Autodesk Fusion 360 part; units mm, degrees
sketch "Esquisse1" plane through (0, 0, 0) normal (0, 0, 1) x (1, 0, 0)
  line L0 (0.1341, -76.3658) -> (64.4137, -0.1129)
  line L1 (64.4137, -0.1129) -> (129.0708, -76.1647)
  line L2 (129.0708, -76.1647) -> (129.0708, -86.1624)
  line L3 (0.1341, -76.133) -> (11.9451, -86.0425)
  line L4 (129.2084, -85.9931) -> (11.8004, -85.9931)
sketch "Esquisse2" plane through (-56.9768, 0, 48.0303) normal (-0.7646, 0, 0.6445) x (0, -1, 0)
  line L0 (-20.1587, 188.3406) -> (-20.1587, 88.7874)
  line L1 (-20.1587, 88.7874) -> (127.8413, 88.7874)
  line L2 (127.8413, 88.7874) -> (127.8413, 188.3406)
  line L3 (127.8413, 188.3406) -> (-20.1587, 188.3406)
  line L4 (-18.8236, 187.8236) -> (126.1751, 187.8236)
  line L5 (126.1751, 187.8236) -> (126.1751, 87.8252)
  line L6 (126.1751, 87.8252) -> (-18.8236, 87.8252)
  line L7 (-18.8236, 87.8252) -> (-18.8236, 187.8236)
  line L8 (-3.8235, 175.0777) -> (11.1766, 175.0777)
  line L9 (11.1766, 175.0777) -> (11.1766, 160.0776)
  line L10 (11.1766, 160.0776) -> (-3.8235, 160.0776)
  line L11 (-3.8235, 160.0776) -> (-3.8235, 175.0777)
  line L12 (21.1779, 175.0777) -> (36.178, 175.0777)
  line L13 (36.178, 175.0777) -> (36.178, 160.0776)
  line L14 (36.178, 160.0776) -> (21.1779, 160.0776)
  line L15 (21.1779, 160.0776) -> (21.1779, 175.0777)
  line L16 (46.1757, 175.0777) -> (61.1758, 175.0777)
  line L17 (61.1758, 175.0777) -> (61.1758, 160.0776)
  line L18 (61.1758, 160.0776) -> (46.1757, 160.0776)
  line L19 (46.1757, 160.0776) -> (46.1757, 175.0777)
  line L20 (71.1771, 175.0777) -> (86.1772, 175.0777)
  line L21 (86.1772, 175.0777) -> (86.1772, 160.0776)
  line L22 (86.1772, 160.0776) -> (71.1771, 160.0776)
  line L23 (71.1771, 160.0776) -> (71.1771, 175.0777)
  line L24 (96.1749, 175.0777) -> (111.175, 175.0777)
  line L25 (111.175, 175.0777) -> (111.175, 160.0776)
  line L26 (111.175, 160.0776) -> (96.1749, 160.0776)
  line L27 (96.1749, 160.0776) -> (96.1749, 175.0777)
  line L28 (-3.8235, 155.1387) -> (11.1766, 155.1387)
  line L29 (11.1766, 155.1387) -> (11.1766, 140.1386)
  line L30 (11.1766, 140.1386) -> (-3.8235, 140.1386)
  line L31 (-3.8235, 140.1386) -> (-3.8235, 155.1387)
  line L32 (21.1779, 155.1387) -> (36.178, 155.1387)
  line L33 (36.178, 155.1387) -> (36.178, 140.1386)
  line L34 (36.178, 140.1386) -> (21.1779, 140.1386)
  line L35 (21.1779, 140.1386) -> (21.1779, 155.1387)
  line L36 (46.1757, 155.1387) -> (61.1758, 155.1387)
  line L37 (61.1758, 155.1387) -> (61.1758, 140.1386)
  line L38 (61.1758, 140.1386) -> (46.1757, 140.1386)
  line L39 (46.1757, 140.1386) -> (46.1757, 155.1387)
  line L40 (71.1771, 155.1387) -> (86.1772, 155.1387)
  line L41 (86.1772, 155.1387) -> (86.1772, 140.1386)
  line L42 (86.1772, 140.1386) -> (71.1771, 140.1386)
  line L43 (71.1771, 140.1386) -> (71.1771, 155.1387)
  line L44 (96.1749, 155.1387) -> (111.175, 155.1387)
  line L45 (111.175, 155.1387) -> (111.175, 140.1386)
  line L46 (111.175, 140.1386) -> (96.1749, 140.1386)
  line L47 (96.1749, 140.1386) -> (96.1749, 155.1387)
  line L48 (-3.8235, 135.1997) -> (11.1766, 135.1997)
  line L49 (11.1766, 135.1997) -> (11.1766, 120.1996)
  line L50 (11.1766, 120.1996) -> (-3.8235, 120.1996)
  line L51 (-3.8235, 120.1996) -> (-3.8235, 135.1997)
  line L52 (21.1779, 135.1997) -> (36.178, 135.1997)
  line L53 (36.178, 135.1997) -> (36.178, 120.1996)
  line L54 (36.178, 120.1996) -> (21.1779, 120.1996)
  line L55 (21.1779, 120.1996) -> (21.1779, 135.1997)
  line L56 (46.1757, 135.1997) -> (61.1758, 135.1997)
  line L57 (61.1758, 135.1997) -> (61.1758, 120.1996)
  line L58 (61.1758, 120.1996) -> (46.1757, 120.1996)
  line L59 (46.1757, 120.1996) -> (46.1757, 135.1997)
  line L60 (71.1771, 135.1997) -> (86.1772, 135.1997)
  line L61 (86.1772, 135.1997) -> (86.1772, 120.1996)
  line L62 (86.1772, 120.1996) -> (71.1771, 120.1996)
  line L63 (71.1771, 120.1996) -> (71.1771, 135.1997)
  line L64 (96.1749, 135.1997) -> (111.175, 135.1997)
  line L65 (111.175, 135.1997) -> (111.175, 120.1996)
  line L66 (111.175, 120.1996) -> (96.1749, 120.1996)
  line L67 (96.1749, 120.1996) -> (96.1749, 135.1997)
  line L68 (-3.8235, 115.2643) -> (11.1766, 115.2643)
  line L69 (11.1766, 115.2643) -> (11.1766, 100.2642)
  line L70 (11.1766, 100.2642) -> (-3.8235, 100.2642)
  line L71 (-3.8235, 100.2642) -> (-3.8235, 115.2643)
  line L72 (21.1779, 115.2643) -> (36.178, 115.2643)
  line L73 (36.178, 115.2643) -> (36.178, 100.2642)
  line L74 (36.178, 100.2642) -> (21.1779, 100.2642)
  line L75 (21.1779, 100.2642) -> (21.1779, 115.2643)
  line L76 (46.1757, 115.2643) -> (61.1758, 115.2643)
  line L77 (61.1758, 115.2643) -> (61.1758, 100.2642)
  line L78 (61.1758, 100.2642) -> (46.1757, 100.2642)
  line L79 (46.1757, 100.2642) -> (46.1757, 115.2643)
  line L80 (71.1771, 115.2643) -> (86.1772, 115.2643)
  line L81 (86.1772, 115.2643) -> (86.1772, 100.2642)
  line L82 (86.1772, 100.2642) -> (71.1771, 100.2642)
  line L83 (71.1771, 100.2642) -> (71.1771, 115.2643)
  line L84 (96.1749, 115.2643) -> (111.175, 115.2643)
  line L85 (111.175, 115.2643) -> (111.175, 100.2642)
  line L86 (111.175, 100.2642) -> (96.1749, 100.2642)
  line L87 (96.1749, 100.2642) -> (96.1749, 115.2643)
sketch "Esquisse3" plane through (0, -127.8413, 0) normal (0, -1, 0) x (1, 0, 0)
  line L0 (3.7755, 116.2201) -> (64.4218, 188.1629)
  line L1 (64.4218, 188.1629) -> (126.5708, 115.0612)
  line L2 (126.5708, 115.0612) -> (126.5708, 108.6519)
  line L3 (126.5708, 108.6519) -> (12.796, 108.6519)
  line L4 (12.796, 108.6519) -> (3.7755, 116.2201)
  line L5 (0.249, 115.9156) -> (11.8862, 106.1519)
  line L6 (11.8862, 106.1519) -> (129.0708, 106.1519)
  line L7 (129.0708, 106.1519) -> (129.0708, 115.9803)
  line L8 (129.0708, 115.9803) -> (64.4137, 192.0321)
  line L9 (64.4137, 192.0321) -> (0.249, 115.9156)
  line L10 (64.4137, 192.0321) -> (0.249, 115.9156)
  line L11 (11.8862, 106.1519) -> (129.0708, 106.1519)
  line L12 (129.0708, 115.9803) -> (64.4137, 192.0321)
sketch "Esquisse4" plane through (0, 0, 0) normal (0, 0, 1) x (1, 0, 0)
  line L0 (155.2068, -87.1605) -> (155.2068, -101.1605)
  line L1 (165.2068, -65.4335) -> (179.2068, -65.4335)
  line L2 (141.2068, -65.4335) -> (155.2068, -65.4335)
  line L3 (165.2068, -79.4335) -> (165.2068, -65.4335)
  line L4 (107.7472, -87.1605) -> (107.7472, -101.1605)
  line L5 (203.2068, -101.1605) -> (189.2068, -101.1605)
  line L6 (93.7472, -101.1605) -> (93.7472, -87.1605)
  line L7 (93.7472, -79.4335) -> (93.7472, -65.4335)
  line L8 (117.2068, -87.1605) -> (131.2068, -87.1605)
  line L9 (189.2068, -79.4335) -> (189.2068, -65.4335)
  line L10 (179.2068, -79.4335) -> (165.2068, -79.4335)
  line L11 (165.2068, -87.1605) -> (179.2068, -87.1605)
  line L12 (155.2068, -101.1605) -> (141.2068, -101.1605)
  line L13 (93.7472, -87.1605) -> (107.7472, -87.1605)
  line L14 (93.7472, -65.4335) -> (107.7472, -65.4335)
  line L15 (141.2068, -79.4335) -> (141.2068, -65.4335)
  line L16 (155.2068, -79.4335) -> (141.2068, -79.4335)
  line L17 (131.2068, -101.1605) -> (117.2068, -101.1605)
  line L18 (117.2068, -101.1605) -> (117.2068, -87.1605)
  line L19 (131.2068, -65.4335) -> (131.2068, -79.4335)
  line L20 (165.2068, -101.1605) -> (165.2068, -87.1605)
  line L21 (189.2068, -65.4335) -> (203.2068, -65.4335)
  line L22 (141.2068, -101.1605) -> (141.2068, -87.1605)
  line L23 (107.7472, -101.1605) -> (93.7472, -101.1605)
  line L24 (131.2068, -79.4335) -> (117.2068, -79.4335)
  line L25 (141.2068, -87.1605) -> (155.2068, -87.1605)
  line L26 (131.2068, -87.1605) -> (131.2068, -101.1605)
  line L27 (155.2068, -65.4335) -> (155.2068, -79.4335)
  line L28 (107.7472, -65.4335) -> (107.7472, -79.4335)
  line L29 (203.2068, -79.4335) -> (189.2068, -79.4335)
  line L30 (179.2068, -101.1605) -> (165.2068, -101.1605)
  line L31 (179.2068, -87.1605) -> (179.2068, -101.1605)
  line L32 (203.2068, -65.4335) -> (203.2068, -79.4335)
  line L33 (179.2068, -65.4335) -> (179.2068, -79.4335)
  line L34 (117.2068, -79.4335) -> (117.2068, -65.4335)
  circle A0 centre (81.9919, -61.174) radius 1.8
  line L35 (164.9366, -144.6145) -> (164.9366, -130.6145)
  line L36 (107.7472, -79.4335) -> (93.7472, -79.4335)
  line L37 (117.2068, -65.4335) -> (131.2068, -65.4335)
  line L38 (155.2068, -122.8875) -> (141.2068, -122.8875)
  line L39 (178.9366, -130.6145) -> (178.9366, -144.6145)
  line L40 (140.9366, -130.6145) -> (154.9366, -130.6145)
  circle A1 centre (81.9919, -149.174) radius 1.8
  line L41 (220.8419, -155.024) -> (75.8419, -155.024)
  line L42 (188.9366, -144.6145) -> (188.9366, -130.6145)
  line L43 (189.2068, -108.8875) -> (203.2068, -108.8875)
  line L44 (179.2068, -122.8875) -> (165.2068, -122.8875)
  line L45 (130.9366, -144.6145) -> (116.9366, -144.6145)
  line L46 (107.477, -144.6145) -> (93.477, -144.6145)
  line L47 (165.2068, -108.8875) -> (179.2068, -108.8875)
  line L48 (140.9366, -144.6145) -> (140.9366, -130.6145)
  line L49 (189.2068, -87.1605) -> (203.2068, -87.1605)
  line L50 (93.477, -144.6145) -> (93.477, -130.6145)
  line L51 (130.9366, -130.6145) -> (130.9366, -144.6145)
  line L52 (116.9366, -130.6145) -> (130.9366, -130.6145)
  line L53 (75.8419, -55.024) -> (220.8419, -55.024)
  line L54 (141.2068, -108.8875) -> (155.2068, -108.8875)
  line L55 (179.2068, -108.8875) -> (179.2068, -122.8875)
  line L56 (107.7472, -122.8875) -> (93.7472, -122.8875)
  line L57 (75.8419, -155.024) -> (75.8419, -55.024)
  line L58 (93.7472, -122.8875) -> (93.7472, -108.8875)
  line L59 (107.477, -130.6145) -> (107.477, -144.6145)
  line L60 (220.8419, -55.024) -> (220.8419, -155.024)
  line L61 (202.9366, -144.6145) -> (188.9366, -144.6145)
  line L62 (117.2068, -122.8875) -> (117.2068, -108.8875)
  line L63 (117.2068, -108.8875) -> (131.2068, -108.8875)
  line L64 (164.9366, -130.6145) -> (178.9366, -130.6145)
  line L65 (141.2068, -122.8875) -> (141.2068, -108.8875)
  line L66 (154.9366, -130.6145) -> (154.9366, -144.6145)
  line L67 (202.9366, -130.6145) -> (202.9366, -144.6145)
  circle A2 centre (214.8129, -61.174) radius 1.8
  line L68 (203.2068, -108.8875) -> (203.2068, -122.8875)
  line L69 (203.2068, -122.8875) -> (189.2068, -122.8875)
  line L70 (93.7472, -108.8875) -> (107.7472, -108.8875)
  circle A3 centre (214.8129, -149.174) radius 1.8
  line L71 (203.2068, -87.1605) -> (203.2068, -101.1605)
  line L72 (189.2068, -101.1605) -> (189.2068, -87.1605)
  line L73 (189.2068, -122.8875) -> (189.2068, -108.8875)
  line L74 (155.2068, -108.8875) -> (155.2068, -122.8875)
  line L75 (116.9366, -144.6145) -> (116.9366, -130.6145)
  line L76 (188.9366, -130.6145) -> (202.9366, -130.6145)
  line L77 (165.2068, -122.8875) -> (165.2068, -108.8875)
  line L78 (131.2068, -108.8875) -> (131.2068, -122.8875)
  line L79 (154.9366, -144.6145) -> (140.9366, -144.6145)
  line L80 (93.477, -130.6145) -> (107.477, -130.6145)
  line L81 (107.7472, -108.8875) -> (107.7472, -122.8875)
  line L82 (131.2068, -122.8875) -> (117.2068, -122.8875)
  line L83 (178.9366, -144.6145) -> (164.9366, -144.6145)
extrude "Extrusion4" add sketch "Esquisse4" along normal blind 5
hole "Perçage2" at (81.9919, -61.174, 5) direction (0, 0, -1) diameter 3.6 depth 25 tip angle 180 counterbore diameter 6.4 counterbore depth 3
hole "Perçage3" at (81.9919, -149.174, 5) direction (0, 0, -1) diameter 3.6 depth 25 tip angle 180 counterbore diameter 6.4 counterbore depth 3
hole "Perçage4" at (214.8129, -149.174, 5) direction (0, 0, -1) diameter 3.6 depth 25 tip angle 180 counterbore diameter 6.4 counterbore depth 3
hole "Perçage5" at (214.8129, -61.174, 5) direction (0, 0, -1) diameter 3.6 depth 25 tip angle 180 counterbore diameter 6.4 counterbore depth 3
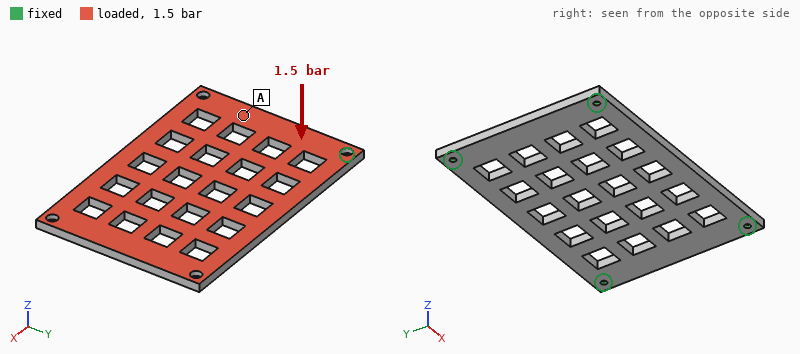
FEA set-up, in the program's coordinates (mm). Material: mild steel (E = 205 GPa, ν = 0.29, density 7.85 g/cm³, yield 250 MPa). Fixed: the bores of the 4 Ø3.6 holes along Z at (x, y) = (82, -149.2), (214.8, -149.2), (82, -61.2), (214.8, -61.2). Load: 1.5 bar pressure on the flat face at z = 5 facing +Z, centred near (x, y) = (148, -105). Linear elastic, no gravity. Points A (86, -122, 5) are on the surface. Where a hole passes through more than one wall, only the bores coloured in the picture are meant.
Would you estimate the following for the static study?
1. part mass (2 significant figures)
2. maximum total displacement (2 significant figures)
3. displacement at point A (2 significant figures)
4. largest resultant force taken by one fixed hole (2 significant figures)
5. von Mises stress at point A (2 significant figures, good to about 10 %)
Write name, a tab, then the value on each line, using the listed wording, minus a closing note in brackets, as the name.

part mass	410 g
maximum total displacement	0.16 mm
displacement at point A	0.034 mm
largest resultant force taken by one fixed hole	900 N
von Mises stress at point A	25 MPa
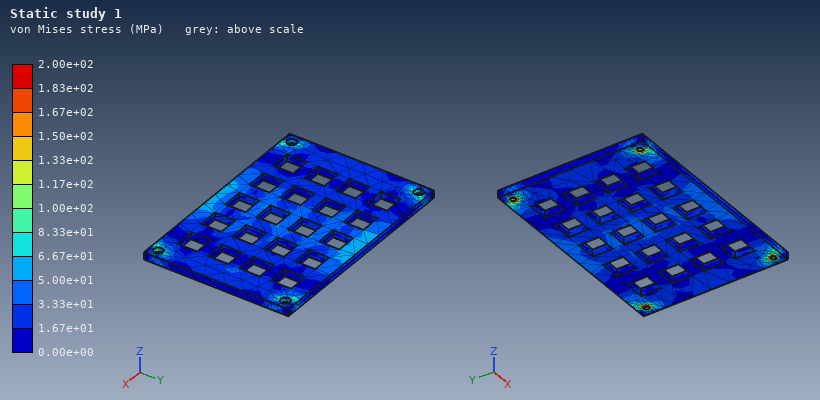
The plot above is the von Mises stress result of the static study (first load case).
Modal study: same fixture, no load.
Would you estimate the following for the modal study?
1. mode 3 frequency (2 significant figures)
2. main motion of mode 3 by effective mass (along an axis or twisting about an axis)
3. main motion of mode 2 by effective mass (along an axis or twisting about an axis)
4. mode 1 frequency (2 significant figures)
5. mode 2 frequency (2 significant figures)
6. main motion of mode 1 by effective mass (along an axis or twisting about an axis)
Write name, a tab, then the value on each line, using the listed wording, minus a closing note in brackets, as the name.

mode 3 frequency	2200 Hz
main motion of mode 3 by effective mass	twisting about Y
main motion of mode 2 by effective mass	twisting about X
mode 1 frequency	910 Hz
mode 2 frequency	1600 Hz
main motion of mode 1 by effective mass	along Z
